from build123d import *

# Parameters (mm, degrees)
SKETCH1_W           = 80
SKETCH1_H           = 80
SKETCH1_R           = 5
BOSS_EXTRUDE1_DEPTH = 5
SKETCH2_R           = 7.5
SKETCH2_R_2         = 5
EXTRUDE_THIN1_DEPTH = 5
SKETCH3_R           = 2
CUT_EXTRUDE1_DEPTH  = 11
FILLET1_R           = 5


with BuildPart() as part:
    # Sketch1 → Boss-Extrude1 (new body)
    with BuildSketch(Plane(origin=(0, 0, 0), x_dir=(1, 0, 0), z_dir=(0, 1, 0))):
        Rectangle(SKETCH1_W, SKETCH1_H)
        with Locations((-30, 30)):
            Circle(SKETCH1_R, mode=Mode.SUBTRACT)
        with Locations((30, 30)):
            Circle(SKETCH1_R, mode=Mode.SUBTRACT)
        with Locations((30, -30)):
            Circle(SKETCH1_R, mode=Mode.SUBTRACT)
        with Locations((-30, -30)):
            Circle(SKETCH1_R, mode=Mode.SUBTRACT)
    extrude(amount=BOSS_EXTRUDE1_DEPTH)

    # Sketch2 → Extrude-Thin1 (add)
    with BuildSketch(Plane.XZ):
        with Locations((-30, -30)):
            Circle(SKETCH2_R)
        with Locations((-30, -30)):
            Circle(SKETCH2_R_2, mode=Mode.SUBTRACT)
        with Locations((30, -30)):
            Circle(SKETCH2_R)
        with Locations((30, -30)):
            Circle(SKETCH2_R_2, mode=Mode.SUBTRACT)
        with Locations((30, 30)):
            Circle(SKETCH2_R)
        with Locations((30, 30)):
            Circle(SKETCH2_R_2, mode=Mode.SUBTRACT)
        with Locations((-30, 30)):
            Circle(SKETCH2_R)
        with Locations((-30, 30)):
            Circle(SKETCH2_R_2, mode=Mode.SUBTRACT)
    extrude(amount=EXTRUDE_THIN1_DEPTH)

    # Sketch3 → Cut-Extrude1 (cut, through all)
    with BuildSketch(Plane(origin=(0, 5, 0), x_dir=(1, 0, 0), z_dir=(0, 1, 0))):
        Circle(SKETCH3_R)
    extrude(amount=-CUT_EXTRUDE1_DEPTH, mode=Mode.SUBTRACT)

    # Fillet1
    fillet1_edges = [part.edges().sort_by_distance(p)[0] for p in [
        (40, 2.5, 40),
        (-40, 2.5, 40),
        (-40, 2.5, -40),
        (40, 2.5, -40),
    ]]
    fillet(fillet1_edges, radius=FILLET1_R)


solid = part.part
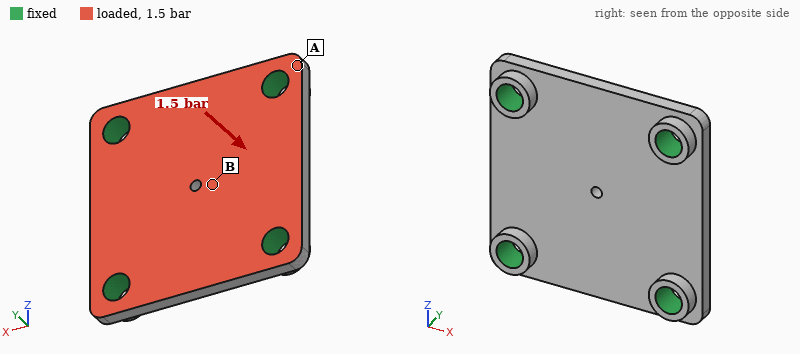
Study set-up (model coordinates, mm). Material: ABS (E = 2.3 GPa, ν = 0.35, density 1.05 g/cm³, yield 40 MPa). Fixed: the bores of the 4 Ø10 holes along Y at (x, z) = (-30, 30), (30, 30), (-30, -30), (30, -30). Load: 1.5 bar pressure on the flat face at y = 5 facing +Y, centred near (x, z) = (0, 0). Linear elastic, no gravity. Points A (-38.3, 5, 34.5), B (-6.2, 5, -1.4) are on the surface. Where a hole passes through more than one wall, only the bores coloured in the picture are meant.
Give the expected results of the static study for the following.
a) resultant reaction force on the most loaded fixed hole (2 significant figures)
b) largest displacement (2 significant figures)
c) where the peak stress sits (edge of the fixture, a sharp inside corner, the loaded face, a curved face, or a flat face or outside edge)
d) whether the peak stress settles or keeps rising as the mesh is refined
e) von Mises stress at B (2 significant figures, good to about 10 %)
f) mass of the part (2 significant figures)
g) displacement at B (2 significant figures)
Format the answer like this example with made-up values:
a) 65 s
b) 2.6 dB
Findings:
a) 230 N
b) 0.32 mm
c) edge of the fixture
d) keeps rising
e) 4.9 MPa
f) 34 g
g) 0.30 mm
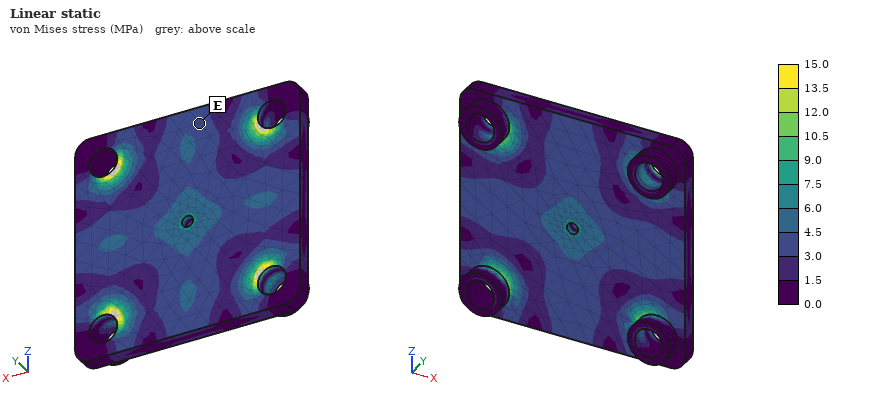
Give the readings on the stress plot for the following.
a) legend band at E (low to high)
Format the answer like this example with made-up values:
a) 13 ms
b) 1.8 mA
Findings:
a) 3.0 to 4.5 MPa
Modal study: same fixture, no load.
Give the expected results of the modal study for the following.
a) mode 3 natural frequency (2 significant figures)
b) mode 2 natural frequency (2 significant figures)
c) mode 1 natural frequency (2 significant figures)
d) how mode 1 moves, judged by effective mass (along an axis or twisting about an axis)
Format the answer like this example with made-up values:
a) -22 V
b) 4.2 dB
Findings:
a) 2900 Hz
b) 2900 Hz
c) 1900 Hz
d) along Y
